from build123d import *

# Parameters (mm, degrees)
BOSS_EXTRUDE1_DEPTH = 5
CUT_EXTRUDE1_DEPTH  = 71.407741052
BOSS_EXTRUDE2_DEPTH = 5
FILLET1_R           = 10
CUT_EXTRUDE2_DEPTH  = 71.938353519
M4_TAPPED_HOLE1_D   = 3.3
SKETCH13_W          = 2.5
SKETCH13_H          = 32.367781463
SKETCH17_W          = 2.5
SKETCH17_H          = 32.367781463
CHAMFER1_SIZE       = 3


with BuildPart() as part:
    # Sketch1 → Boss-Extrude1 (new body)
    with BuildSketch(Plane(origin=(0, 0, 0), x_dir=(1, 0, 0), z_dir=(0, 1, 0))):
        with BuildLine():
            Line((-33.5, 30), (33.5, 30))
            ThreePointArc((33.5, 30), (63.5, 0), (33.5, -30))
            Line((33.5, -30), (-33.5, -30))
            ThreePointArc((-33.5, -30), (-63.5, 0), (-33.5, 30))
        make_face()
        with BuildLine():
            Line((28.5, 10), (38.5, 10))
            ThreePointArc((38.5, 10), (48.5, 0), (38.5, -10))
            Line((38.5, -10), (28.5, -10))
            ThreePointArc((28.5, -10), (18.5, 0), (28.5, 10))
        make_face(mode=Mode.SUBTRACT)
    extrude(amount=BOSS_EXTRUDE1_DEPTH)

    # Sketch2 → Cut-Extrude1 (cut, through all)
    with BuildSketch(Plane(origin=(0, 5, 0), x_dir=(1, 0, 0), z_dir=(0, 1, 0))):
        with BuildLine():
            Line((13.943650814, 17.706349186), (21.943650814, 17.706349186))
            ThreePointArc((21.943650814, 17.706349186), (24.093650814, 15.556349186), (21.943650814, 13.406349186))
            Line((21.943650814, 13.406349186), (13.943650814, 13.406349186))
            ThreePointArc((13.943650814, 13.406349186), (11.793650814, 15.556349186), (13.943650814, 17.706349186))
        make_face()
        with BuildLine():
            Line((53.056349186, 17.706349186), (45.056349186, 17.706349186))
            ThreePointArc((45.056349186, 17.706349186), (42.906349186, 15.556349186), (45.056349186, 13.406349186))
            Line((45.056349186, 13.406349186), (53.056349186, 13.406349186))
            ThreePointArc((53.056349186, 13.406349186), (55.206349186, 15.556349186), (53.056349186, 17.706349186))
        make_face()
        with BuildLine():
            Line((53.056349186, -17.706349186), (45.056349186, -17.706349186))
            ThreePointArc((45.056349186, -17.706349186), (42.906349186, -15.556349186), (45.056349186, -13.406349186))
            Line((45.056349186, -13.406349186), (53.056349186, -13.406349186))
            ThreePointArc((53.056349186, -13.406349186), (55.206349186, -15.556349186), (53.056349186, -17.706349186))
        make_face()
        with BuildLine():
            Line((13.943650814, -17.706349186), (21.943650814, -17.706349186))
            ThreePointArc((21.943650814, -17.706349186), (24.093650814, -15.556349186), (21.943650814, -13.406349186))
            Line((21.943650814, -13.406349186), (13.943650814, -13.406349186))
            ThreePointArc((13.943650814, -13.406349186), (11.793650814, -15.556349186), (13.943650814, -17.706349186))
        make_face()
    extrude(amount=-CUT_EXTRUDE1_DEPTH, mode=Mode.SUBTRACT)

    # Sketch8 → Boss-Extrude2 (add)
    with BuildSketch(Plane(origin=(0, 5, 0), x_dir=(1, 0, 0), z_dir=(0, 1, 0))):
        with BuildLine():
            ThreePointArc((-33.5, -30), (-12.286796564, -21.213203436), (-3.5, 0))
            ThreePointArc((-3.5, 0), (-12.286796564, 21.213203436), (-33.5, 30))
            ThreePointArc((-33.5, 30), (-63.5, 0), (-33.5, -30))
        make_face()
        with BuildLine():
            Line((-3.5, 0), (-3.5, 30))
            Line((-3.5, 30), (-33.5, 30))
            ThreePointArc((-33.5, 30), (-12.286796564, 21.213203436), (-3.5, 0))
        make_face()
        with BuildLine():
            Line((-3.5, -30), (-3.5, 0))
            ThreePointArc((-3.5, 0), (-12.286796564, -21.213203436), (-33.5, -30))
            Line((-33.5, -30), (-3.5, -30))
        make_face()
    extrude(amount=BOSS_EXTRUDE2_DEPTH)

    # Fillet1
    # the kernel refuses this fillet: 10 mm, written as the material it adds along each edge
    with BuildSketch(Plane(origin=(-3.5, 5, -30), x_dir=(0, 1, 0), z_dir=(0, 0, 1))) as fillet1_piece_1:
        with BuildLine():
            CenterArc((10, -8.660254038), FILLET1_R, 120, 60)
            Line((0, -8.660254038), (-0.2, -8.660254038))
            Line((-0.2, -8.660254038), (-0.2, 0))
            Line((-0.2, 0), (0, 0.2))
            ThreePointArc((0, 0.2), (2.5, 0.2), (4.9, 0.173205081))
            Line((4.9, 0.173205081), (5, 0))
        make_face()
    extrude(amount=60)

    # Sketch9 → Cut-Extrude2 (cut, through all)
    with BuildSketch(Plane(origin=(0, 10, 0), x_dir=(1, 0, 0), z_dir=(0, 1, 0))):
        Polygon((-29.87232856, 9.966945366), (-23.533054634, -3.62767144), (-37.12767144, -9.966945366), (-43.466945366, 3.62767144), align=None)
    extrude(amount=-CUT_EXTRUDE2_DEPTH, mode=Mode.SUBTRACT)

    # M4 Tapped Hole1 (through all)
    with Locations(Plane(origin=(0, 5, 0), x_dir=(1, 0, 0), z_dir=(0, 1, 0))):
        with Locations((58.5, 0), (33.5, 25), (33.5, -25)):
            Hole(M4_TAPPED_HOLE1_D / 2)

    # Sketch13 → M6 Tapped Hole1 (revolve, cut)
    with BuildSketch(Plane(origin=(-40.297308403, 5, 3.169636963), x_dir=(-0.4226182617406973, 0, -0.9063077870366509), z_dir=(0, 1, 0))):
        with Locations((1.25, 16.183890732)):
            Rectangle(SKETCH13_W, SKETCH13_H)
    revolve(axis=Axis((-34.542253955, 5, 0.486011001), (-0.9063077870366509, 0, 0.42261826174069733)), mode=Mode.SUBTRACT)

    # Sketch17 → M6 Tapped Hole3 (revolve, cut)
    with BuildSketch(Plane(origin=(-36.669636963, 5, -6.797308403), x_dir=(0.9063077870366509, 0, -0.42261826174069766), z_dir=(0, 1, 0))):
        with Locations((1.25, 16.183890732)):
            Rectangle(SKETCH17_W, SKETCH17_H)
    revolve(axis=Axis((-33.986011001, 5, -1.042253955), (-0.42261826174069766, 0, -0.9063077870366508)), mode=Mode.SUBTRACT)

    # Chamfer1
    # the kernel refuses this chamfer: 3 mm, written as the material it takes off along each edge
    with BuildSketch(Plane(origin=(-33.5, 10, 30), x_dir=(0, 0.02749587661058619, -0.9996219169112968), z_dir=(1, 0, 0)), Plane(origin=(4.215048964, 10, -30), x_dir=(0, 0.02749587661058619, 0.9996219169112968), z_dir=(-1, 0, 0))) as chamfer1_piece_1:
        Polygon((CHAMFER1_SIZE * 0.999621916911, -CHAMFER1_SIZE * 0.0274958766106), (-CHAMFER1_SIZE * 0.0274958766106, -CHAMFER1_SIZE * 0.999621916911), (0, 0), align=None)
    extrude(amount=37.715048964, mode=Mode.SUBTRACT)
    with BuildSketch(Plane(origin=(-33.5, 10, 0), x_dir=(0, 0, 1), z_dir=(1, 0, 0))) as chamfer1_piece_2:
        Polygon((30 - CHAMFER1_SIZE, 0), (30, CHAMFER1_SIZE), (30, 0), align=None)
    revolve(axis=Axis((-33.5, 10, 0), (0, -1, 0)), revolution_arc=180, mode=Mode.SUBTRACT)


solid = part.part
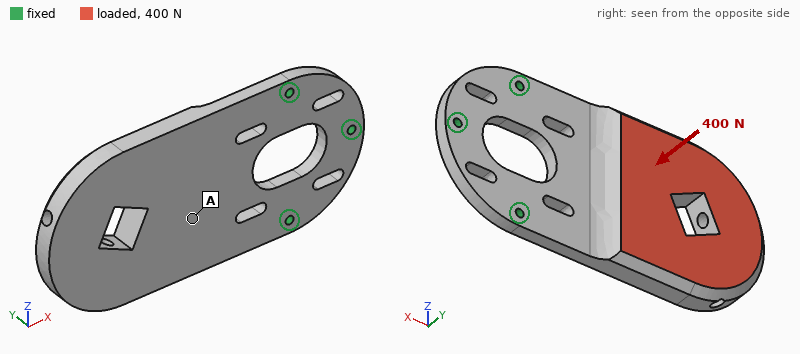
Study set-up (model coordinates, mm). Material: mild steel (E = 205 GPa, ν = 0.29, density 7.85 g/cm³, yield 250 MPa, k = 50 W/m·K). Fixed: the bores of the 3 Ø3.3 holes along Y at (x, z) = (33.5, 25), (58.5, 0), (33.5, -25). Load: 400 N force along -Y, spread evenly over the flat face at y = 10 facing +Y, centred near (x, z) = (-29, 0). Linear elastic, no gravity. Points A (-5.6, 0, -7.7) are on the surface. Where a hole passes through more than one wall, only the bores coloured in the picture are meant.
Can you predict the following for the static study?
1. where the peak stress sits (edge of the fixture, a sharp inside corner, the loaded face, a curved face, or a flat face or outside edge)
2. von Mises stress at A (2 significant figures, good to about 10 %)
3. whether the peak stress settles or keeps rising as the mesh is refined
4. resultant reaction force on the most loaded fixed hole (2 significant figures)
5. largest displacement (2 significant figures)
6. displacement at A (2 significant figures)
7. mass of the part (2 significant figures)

edge of the fixture
18 MPa
keeps rising
330 N
0.61 mm
0.19 mm
340 g
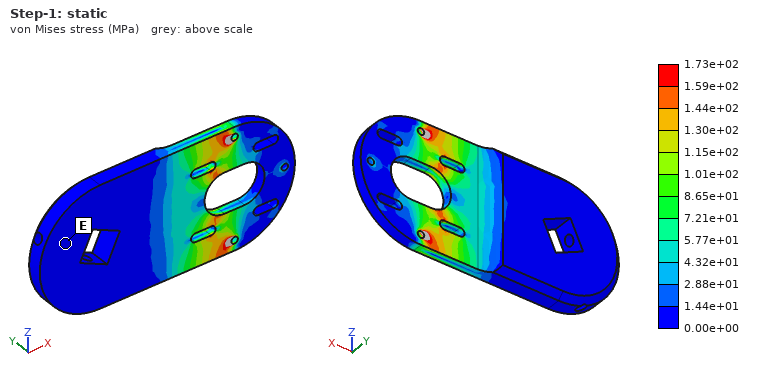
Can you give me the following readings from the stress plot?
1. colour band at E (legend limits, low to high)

0.00e+00 to 1.44e+01 MPa
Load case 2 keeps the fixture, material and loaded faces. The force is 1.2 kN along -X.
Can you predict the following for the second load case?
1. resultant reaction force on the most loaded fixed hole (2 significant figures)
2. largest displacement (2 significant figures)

550 N
0.28 mm
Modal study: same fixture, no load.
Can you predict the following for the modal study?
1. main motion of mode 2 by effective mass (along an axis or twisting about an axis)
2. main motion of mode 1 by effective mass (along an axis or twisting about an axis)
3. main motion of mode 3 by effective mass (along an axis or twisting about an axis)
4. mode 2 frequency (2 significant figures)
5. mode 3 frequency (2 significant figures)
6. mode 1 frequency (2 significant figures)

twisting about X
along Y
along Z
1900 Hz
3300 Hz
330 Hz
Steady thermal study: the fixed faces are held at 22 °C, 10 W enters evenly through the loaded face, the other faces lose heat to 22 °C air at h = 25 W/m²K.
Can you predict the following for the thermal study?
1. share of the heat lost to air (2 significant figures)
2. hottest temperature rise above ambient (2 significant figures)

50 %
26 K
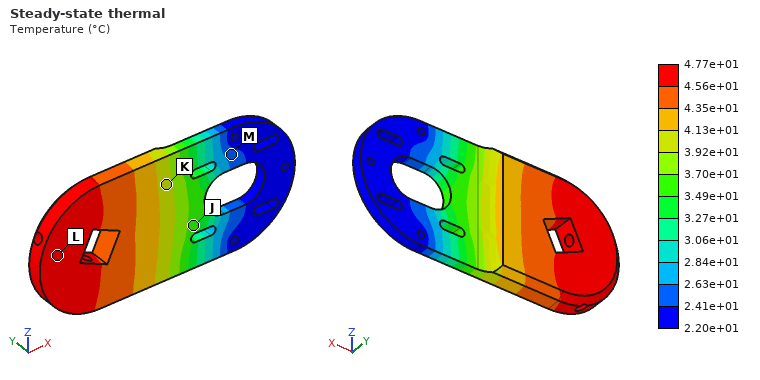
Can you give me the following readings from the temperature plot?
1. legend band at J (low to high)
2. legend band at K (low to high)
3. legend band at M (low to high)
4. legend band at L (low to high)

3.49e+01 to 3.70e+01 °C
3.92e+01 to 4.13e+01 °C
2.41e+01 to 2.63e+01 °C
4.56e+01 to 4.77e+01 °C
